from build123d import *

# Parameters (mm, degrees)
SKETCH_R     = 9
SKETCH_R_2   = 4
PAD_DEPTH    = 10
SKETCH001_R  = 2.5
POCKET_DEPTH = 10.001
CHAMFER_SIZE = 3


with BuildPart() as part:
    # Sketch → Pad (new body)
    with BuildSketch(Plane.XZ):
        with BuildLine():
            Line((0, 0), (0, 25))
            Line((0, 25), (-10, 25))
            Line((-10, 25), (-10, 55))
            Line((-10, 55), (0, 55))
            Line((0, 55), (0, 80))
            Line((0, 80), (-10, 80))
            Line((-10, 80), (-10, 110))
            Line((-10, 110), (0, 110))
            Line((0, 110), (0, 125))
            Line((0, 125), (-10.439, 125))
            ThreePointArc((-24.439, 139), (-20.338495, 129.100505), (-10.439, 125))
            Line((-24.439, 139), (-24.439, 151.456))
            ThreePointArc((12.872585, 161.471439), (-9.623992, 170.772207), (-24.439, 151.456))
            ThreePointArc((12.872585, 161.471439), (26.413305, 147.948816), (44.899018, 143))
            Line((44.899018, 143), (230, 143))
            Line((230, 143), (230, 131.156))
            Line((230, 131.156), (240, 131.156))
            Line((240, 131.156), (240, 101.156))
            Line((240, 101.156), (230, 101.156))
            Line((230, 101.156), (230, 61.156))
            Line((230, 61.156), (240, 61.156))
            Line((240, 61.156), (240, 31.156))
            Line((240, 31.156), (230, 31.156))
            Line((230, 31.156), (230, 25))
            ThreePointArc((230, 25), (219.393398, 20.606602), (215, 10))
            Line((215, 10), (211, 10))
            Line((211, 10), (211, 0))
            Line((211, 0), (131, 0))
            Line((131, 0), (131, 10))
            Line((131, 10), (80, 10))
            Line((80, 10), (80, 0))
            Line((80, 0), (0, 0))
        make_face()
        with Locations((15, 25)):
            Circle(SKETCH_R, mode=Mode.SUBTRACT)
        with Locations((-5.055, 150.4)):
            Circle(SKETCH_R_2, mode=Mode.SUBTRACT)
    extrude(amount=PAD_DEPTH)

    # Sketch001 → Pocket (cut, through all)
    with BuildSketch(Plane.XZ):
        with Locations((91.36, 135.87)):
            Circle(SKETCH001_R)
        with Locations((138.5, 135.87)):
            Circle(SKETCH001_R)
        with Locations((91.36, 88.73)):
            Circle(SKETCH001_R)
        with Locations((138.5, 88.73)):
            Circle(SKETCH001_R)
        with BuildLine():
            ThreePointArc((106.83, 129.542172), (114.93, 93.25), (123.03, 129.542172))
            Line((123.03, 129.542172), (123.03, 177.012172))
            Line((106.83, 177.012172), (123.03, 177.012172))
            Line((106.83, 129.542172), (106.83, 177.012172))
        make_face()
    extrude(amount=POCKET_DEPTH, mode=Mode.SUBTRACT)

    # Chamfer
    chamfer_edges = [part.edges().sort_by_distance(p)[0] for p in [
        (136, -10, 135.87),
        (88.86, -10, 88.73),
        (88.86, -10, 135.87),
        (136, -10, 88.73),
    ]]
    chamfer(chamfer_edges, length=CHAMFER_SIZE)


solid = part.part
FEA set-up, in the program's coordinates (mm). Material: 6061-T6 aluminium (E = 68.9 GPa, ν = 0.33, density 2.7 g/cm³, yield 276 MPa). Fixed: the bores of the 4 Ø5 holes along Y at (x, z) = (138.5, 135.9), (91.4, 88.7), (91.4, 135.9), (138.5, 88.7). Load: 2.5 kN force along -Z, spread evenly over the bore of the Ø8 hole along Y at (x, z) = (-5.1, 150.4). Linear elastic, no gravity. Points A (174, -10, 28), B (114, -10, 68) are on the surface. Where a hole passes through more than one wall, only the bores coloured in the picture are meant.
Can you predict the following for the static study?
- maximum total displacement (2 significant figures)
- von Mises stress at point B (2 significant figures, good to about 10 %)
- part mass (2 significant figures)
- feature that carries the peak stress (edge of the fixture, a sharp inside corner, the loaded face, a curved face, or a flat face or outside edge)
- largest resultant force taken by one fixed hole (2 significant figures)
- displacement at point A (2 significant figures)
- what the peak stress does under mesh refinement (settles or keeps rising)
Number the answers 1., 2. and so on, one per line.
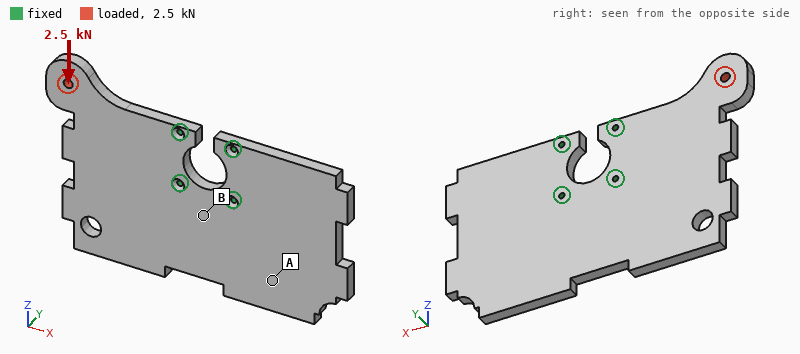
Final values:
1. 69 µm
2. 5.5 MPa
3. 890 g
4. edge of the fixture
5. 3.2 kN
6. 11 µm
7. keeps rising
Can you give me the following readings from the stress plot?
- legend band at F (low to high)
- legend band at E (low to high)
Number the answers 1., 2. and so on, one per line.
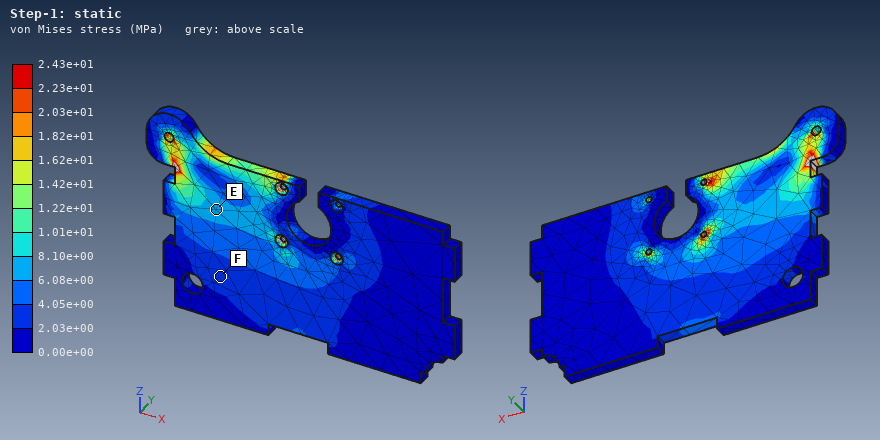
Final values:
1. 2.03e+00 to 4.05e+00 MPa
2. 6.08e+00 to 8.10e+00 MPa
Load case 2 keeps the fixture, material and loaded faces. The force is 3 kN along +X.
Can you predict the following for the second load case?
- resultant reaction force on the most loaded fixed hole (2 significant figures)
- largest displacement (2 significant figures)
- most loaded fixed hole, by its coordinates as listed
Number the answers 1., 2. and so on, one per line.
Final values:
1. 2.9 kN
2. 59 µm
3. (91.4, 135.9)
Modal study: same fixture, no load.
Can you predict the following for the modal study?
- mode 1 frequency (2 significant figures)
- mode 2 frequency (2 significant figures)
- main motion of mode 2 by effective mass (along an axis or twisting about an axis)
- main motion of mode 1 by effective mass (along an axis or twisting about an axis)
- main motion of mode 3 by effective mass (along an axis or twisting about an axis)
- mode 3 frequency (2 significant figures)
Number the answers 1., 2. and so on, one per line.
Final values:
1. 560 Hz
2. 650 Hz
3. along Y
4. along Y
5. twisting about X
6. 740 Hz
